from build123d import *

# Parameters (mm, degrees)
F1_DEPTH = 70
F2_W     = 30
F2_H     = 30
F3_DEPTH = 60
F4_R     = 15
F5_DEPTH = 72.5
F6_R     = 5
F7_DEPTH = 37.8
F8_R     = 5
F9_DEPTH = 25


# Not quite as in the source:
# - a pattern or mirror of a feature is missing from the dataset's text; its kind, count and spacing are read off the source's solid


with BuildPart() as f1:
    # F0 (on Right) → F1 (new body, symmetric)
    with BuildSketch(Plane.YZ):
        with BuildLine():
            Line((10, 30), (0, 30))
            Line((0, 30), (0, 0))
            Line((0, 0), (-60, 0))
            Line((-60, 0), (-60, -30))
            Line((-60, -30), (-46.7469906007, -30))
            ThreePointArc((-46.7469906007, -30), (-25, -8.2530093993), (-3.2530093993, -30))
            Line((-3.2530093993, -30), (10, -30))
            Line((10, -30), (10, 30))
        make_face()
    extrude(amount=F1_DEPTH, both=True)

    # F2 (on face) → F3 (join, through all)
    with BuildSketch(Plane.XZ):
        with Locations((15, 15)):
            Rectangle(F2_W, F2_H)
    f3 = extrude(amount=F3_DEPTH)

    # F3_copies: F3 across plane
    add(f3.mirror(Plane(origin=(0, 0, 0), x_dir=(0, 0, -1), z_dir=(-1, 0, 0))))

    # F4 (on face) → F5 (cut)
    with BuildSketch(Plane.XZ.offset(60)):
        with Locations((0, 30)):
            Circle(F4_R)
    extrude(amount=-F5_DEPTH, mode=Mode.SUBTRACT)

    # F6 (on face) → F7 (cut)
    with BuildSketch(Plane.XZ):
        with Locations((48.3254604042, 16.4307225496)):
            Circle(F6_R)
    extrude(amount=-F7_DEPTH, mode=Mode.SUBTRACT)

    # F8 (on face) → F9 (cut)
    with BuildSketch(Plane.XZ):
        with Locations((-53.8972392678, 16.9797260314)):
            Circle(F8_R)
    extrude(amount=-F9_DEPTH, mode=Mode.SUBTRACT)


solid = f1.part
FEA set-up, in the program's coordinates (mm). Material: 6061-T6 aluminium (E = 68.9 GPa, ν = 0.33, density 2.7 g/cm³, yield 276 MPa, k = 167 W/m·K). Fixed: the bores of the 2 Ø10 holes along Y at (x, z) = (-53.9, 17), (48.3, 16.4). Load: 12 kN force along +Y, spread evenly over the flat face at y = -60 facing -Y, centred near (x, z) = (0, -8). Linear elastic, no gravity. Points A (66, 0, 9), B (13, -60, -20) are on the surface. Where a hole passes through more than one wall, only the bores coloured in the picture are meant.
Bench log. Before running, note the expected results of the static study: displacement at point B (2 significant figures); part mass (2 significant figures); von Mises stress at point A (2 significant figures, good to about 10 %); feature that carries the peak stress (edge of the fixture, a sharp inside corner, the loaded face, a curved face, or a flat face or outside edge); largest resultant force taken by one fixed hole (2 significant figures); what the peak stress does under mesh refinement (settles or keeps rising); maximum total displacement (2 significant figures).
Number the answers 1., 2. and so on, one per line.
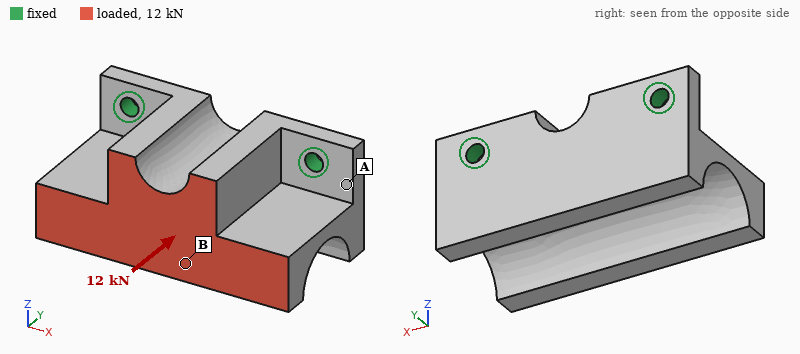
1. 0.35 mm
2. 850 g
3. 63 MPa
4. edge of the fixture
5. 6.3 kN
6. keeps rising
7. 0.39 mm
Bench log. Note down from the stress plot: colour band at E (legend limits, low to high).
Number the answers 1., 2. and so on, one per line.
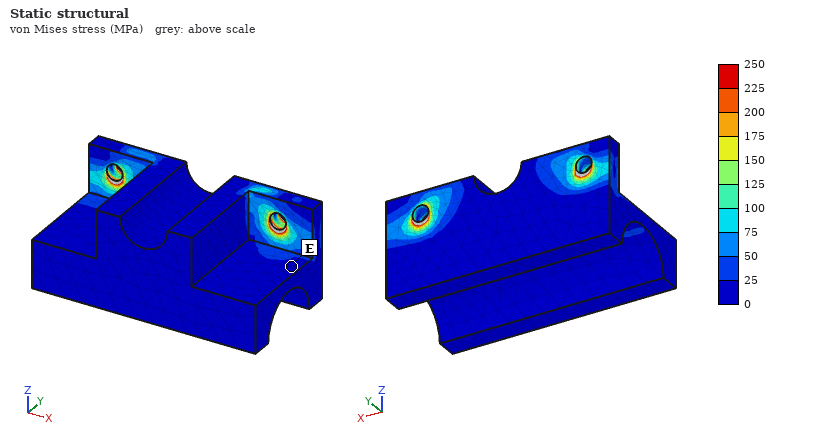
1. 0 to 25 MPa
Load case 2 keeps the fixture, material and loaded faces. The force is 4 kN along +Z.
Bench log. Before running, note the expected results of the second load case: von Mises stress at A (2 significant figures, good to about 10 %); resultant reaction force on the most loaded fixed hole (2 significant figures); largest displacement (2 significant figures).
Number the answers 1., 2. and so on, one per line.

1. 70 MPa
2. 2.8 kN
3. 0.45 mm
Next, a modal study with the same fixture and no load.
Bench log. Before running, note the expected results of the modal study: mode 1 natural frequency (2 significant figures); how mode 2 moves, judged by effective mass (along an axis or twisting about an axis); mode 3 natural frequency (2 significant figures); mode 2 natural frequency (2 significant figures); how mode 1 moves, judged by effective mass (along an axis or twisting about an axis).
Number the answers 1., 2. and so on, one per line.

1. 900 Hz
2. along X
3. 3600 Hz
4. 3100 Hz
5. along Z
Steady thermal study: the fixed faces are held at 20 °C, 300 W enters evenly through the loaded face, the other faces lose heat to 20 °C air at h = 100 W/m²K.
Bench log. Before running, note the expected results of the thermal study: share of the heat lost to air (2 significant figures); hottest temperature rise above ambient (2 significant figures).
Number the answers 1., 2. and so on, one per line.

1. 42 %
2. 54 K
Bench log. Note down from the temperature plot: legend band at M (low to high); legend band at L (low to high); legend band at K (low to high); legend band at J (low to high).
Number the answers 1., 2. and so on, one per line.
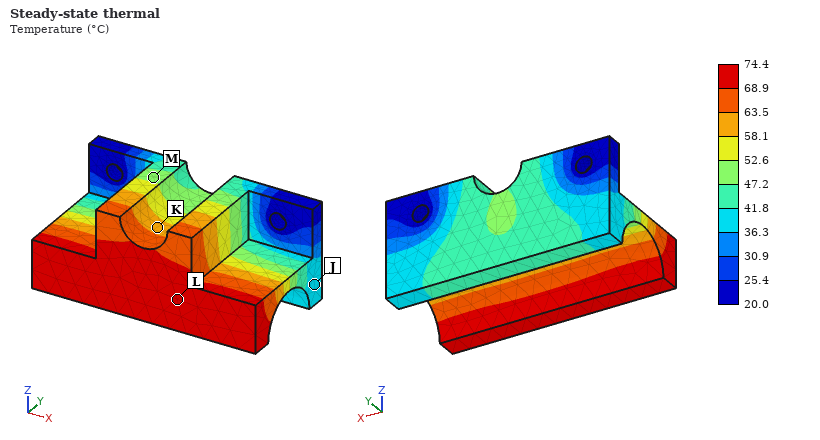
1. 47.2 to 52.6 °C
2. 68.9 to 74.4 °C
3. 58.1 to 63.5 °C
4. 36.3 to 41.8 °C
